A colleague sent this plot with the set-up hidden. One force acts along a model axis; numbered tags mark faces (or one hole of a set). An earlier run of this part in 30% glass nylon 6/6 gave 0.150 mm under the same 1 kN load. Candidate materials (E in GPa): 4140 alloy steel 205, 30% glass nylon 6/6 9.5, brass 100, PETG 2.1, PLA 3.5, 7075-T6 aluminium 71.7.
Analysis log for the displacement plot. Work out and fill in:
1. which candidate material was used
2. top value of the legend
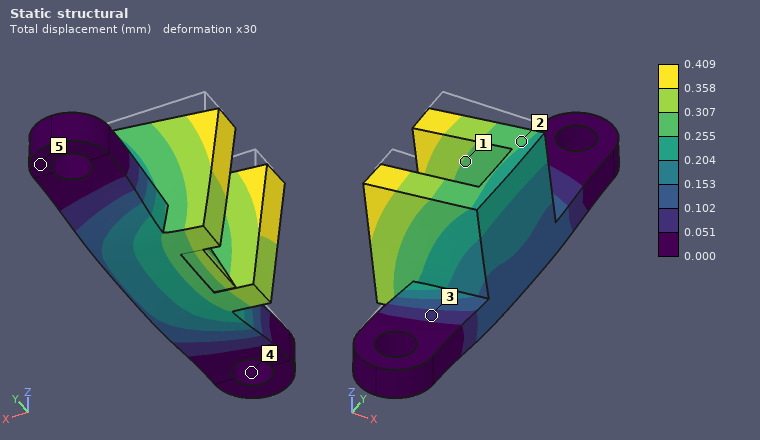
PLA
0.409 mm
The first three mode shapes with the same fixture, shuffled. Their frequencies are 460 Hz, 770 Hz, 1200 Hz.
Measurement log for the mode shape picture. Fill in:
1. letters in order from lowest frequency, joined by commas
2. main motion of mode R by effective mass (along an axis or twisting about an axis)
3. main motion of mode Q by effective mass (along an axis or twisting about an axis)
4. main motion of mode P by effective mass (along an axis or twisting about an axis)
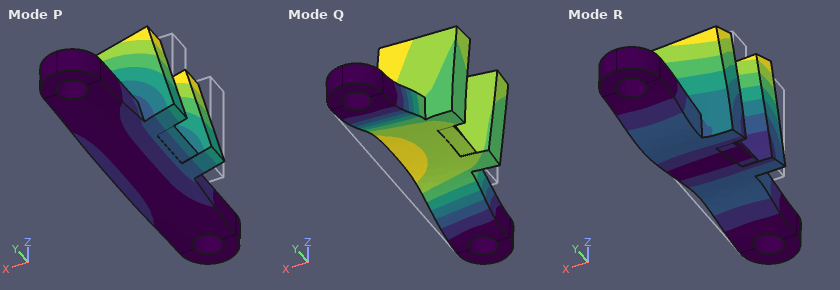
P, Q, R
along Y
along Z
along X
